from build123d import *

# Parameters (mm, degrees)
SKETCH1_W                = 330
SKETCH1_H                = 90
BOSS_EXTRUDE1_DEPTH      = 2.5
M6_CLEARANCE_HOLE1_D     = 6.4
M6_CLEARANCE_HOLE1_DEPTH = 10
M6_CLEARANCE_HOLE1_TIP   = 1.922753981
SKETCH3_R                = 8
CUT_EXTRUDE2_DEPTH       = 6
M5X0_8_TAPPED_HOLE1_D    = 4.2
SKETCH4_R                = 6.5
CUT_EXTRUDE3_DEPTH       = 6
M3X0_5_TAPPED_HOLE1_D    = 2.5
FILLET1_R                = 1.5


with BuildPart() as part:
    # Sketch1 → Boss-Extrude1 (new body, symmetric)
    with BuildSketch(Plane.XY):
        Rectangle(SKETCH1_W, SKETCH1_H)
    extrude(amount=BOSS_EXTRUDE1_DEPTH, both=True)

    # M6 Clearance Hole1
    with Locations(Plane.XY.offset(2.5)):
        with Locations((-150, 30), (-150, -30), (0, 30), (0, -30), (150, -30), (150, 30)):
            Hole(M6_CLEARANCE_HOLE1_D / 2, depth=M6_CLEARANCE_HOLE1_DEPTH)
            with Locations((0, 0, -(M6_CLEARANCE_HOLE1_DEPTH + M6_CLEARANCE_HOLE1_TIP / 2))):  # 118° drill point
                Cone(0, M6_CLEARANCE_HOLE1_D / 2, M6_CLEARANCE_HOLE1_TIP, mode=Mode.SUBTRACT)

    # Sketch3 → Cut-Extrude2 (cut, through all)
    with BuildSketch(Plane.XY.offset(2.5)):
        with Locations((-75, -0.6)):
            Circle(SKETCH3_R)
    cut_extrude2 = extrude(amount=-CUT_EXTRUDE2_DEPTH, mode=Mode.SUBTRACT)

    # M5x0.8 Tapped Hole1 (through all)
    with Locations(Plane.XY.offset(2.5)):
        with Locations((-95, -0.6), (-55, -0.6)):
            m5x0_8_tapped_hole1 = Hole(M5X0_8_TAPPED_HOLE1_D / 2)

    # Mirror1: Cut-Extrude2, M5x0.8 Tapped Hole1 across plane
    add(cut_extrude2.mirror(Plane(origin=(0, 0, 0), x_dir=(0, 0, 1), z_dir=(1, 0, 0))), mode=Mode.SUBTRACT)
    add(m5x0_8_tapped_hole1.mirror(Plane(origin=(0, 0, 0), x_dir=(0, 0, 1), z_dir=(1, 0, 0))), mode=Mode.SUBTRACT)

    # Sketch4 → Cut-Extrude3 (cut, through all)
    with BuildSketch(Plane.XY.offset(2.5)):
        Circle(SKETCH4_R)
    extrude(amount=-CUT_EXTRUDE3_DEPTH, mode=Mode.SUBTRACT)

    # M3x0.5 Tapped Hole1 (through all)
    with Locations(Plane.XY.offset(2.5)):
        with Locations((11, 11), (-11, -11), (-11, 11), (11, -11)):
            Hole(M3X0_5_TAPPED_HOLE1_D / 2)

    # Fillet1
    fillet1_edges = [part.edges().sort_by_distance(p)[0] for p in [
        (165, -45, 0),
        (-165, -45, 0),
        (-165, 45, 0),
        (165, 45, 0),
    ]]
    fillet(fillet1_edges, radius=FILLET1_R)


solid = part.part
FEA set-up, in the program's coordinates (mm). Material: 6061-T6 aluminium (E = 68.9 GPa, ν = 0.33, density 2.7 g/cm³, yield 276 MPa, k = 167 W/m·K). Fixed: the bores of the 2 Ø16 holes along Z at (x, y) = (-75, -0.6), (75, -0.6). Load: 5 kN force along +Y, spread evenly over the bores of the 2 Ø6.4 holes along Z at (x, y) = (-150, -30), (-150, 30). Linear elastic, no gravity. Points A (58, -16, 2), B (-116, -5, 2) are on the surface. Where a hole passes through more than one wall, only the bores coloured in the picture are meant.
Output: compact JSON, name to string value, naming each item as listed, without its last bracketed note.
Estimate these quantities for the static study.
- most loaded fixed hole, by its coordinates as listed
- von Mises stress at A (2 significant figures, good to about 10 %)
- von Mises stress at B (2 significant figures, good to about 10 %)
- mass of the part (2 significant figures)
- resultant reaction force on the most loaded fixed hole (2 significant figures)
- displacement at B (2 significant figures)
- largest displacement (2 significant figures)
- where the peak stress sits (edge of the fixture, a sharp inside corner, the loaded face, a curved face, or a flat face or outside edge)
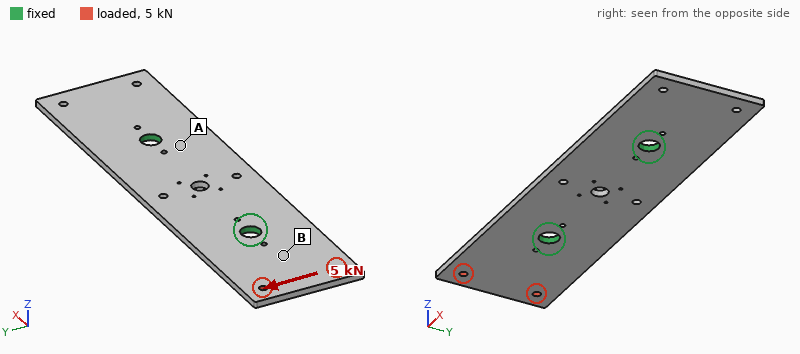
{"most loaded fixed hole, by its coordinates as listed": "(-75, -0.6)", "von Mises stress at A": "10 MPa", "von Mises stress at B": "28 MPa", "mass of the part": "390 g", "resultant reaction force on the most loaded fixed hole": "6.9 kN", "displacement at B": "0.069 mm", "largest displacement": "0.18 mm", "where the peak stress sits": "edge of the fixture"}
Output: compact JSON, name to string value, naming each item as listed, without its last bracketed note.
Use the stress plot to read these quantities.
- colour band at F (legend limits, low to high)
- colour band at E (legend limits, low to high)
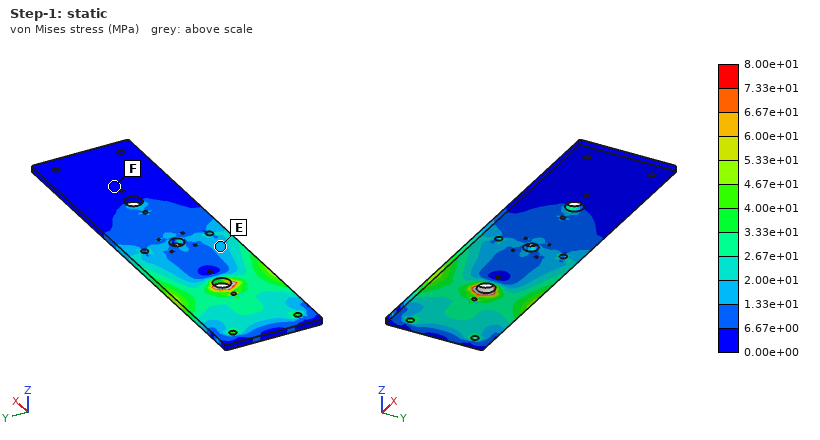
{"colour band at F": "0.00e+00 to 6.67e+00 MPa", "colour band at E": "1.33e+01 to 2.00e+01 MPa"}
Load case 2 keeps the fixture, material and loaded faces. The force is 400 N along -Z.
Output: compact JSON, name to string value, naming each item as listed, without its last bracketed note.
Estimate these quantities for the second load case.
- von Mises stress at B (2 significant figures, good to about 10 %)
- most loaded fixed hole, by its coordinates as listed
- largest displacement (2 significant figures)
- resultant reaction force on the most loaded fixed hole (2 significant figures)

{"von Mises stress at B": "31 MPa", "most loaded fixed hole, by its coordinates as listed": "(-75, -0.6)", "largest displacement": "1.0 mm", "resultant reaction force on the most loaded fixed hole": "420 N"}
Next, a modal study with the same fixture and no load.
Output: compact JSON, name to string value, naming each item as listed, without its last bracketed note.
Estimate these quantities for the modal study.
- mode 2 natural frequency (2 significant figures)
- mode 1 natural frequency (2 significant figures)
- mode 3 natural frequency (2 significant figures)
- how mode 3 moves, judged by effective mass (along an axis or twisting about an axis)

{"mode 2 natural frequency": "530 Hz", "mode 1 natural frequency": "530 Hz", "mode 3 natural frequency": "1000 Hz", "how mode 3 moves, judged by effective mass": "twisting about X"}
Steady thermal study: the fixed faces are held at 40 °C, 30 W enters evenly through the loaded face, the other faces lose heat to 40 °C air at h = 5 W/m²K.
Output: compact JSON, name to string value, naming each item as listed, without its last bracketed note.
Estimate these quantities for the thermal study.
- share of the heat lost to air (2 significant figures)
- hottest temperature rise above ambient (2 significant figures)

{"share of the heat lost to air": "6.6 %", "hottest temperature rise above ambient": "36 K"}
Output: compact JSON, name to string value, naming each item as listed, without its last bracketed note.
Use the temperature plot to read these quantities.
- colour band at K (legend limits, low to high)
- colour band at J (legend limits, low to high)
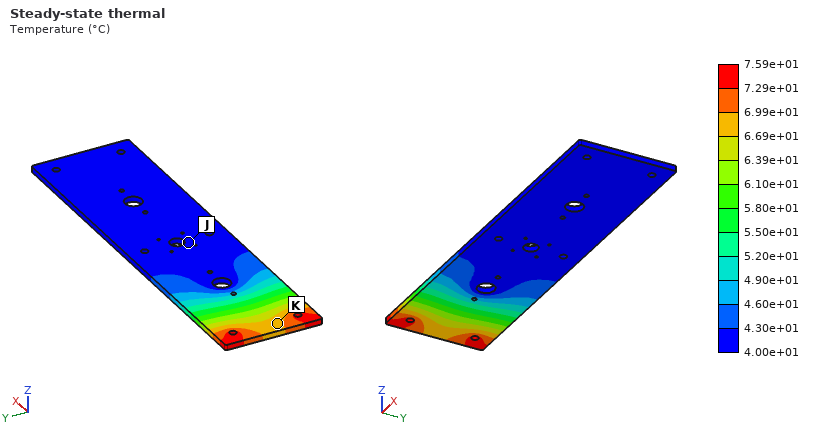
{"colour band at K": "6.69e+01 to 6.99e+01 °C", "colour band at J": "4.00e+01 to 4.30e+01 °C"}
